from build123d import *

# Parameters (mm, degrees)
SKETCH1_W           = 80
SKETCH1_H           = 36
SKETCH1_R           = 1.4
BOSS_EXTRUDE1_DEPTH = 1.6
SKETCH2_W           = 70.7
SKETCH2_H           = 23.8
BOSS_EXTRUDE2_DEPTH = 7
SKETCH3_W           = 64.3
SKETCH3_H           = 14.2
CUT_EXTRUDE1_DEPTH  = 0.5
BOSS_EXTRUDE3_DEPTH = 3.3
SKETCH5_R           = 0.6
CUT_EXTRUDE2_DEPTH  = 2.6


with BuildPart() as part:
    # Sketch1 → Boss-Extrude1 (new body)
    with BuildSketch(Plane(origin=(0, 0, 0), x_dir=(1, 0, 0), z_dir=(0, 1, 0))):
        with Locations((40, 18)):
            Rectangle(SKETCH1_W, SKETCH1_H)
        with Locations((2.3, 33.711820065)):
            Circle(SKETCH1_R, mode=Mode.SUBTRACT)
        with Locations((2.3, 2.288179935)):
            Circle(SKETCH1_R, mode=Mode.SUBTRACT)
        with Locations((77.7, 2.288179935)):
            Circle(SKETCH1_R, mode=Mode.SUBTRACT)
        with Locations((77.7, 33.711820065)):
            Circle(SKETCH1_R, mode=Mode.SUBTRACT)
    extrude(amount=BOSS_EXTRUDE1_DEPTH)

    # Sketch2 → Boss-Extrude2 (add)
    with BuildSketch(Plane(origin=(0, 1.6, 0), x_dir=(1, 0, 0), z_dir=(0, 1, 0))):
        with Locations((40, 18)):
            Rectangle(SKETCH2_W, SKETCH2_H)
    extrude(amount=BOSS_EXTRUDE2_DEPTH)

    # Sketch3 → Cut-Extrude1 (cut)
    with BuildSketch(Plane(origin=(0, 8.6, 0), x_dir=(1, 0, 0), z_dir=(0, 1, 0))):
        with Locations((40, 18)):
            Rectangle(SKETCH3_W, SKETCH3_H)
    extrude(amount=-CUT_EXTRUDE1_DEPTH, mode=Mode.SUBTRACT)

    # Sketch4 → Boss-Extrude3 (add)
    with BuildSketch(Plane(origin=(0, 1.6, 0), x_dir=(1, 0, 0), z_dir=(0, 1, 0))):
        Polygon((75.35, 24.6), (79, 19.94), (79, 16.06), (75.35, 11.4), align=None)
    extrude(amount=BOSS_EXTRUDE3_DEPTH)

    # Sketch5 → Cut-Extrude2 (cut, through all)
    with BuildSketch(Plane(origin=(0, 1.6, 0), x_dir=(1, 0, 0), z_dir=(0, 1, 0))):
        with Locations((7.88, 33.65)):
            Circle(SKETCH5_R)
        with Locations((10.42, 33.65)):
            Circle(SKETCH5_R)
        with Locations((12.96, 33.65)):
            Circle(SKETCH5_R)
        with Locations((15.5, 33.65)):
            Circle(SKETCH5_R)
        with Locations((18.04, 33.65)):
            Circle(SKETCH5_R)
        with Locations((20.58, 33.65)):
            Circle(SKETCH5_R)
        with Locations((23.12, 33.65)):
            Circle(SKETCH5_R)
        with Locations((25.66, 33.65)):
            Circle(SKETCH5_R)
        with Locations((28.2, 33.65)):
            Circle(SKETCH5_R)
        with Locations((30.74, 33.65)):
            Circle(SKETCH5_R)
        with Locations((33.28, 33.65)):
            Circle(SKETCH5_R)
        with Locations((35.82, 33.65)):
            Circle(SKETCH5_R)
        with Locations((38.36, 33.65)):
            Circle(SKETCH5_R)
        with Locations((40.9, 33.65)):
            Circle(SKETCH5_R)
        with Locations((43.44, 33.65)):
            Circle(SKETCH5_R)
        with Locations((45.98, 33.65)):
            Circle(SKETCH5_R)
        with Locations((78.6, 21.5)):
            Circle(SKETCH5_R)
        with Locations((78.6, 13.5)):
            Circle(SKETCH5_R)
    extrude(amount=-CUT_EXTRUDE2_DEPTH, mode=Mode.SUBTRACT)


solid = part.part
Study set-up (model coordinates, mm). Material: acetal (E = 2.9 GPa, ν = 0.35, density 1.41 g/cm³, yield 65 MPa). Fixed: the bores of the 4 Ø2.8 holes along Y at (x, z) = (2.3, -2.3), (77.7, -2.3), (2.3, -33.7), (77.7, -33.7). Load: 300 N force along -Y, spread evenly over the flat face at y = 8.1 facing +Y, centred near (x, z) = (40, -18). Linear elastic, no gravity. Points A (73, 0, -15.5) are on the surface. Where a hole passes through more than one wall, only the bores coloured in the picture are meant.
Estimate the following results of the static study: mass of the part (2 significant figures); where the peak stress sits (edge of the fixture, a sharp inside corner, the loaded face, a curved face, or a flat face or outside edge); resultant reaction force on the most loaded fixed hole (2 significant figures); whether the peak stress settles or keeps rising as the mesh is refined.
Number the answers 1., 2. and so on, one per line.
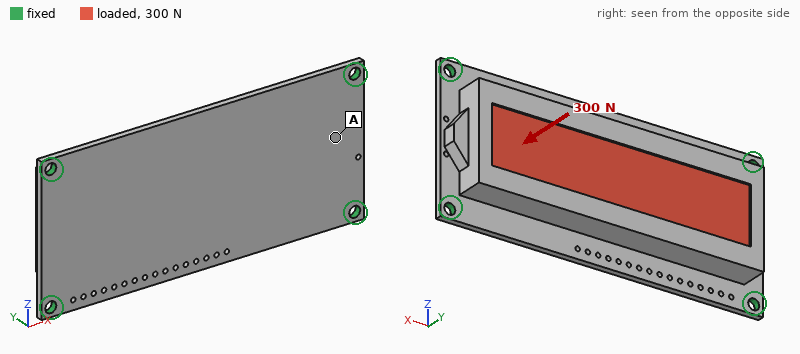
1. 23 g
2. edge of the fixture
3. 150 N
4. keeps rising
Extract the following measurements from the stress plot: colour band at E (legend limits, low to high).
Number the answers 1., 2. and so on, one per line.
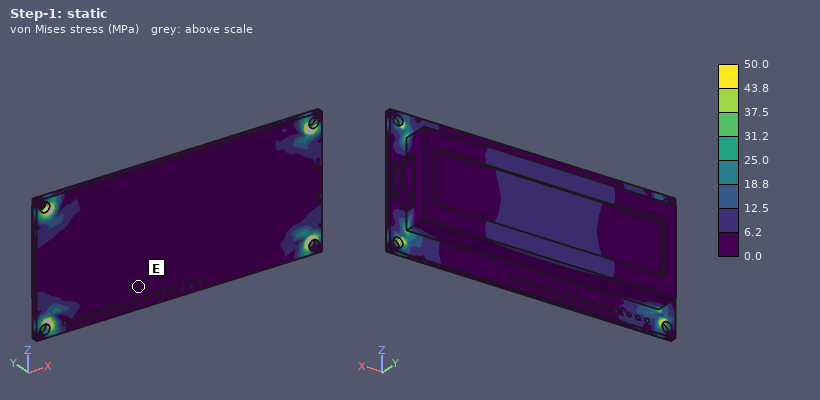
1. 0.0 to 6.2 MPa
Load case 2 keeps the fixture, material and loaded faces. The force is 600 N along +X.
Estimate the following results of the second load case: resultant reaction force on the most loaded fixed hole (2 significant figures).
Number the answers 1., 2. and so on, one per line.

1. 170 N
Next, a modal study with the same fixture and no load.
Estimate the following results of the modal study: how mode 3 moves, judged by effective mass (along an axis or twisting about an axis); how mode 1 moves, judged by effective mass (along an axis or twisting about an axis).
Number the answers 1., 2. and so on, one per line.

1. twisting about Z
2. along Y
